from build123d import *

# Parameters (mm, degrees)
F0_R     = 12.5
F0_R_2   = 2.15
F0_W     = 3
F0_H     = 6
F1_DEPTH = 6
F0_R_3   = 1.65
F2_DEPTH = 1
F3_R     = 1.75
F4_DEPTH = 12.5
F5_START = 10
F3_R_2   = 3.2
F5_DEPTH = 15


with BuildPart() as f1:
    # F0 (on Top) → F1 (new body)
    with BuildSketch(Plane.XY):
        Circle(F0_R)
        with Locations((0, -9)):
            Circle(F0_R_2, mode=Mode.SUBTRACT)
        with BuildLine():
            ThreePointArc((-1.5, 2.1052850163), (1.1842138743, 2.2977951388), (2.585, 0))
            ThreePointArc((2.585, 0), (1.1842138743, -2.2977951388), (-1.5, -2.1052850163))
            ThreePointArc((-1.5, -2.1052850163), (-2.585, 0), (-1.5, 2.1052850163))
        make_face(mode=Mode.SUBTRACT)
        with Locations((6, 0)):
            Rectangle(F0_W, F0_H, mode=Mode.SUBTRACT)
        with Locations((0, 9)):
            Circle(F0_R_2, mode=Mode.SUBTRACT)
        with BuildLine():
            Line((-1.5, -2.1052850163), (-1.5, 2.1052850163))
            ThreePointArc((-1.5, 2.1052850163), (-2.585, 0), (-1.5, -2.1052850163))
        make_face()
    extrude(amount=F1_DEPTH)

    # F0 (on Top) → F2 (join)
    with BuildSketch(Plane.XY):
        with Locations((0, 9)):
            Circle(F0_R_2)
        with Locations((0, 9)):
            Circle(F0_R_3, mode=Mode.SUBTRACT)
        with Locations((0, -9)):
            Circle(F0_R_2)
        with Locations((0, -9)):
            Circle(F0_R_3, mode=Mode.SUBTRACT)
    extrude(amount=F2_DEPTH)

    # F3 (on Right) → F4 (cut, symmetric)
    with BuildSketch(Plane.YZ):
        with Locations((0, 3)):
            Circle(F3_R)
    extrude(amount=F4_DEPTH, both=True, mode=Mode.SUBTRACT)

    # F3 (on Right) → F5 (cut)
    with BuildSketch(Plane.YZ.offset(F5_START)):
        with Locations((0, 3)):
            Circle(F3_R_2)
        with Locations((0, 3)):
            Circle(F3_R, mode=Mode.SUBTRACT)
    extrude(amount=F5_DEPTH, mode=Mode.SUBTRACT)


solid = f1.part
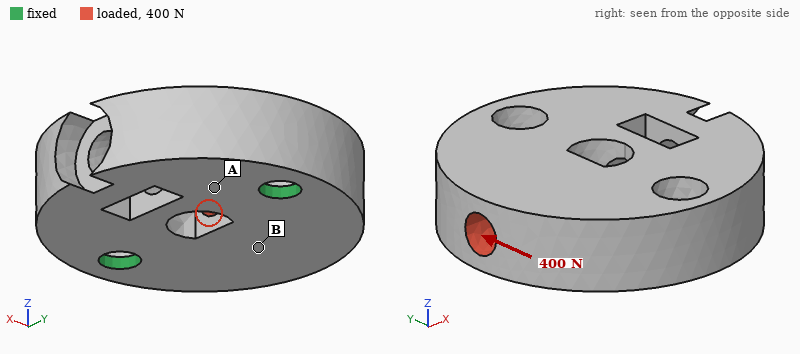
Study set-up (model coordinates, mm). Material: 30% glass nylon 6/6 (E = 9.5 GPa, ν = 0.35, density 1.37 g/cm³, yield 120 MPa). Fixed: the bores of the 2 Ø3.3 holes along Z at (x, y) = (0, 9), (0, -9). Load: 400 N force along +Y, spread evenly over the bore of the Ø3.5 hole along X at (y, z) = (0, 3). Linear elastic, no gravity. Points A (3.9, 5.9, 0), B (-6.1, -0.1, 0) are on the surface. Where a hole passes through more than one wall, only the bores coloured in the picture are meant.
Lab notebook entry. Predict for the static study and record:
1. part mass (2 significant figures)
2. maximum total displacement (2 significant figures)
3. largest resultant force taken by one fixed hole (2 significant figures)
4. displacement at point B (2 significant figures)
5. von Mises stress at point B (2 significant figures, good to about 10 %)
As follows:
3.2 g
23 µm
250 N
17 µm
11 MPa
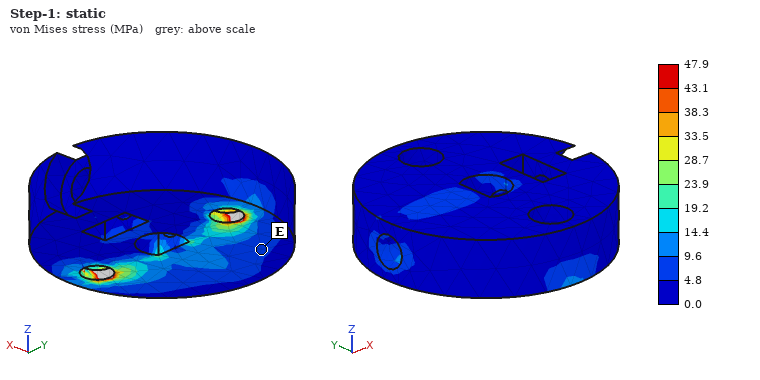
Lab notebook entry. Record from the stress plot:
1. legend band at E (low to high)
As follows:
4.8 to 9.6 MPa
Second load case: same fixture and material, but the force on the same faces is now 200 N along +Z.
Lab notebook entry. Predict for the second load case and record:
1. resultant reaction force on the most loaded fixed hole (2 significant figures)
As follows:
120 N
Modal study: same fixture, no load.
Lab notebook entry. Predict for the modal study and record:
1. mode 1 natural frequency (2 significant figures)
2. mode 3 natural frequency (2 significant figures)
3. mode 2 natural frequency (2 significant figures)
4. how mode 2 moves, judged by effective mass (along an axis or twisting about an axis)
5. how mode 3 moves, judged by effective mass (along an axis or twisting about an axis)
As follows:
4400 Hz
15 kHz
14 kHz
along Z
twisting about Z
